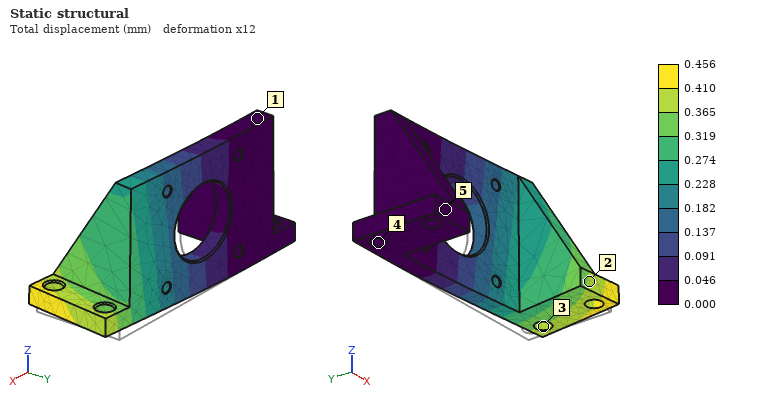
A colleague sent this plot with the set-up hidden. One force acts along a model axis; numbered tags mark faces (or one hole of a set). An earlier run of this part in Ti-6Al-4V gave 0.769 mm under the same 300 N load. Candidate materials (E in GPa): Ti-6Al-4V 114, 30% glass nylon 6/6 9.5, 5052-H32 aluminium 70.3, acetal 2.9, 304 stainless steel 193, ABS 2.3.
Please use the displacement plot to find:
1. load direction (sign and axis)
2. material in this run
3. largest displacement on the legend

-Y
304 stainless steel
0.456 mm
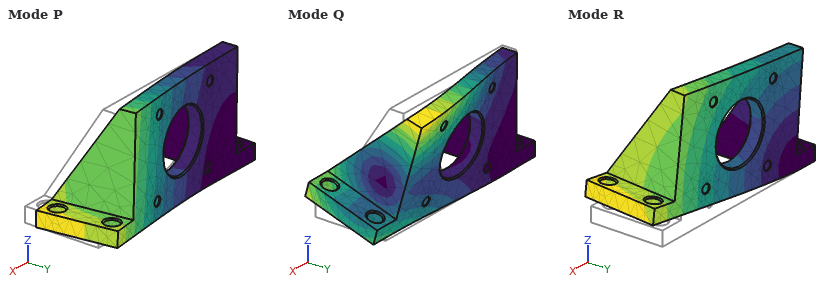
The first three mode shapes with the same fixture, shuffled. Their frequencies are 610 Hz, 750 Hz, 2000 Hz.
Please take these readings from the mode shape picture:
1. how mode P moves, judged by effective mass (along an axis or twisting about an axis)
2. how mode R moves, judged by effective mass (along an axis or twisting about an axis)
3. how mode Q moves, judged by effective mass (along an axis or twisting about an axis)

along Y
along Z
twisting about X
